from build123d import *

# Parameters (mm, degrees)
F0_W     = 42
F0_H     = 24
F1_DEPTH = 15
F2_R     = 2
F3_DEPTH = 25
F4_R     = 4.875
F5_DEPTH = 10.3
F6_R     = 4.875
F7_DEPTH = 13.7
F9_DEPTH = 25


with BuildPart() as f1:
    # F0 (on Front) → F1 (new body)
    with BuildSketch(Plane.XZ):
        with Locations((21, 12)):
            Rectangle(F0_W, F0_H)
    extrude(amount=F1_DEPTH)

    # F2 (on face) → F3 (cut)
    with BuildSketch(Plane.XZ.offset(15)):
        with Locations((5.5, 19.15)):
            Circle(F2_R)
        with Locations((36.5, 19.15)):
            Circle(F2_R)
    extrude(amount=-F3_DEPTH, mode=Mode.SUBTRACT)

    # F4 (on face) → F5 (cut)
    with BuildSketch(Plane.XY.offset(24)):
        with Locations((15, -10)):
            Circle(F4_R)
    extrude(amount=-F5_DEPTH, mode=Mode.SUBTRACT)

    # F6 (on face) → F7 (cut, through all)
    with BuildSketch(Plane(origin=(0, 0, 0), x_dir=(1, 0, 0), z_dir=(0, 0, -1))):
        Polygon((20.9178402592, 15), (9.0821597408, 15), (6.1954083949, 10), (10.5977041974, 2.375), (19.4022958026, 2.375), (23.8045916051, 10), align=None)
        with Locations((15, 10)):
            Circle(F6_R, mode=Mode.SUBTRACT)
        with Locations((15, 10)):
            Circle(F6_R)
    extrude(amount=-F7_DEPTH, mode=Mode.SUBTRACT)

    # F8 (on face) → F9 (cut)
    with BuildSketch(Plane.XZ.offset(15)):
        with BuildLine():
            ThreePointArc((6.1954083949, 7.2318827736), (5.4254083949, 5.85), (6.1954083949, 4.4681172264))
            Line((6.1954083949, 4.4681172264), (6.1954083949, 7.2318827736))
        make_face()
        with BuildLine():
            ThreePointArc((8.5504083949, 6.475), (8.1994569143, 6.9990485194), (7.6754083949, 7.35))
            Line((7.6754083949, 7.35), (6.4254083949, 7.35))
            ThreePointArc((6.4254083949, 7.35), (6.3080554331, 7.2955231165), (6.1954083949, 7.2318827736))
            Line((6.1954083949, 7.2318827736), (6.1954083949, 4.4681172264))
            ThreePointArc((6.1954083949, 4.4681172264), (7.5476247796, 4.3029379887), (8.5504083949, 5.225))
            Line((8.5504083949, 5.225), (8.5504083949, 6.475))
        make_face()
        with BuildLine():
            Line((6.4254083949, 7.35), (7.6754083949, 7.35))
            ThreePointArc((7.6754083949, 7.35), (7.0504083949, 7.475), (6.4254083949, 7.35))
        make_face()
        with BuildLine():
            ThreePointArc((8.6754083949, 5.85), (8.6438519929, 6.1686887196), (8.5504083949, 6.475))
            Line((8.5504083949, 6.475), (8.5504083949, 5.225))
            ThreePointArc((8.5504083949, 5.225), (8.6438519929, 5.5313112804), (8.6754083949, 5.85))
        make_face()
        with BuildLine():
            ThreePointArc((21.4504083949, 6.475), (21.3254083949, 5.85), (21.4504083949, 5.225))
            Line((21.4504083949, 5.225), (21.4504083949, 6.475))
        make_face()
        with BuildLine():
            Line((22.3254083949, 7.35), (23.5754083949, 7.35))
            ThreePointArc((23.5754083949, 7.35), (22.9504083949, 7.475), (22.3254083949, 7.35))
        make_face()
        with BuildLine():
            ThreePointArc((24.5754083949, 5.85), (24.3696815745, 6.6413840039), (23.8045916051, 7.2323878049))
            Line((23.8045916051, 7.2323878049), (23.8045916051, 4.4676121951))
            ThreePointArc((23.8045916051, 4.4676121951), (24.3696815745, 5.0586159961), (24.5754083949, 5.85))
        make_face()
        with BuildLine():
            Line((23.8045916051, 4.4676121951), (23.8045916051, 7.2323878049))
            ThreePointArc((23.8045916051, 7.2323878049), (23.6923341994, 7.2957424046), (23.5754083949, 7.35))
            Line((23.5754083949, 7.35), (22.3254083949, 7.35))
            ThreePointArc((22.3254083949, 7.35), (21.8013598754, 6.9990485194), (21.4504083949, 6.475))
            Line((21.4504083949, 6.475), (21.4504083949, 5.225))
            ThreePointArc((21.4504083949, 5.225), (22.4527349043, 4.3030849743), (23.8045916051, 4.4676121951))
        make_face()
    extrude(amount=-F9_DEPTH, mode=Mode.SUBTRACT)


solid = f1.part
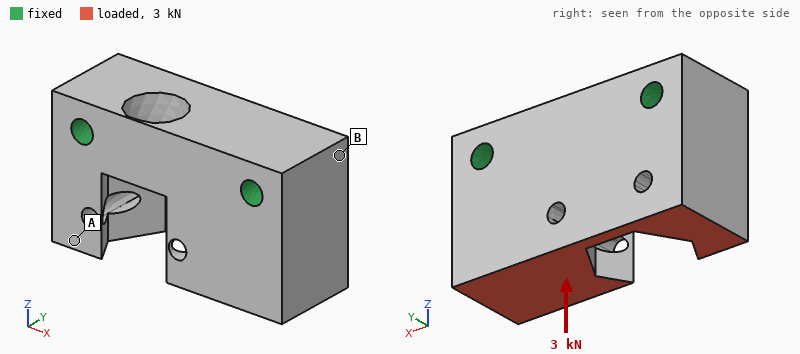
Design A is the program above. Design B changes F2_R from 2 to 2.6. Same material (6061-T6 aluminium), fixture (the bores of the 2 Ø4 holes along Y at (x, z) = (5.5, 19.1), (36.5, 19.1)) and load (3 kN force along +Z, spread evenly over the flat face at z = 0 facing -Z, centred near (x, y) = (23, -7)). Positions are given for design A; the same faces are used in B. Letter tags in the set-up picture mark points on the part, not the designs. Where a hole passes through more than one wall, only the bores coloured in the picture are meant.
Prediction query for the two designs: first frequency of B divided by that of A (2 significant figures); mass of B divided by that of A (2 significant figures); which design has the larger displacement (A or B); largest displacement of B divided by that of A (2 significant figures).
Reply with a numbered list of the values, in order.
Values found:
1. 1.1
2. 0.98
3. A
4. 0.91
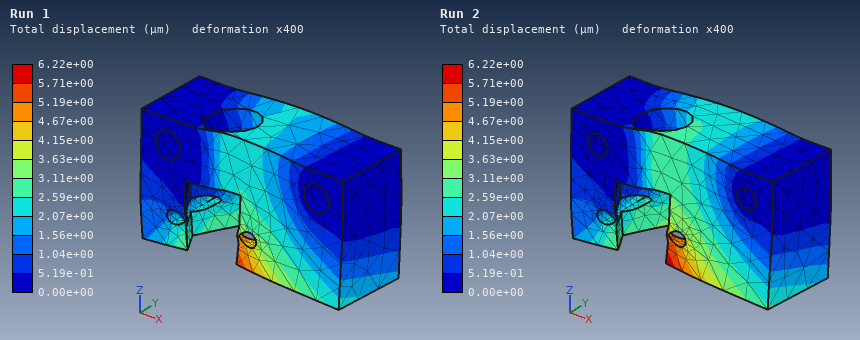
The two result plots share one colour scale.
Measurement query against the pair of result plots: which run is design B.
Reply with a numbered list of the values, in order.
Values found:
1. Run 1
